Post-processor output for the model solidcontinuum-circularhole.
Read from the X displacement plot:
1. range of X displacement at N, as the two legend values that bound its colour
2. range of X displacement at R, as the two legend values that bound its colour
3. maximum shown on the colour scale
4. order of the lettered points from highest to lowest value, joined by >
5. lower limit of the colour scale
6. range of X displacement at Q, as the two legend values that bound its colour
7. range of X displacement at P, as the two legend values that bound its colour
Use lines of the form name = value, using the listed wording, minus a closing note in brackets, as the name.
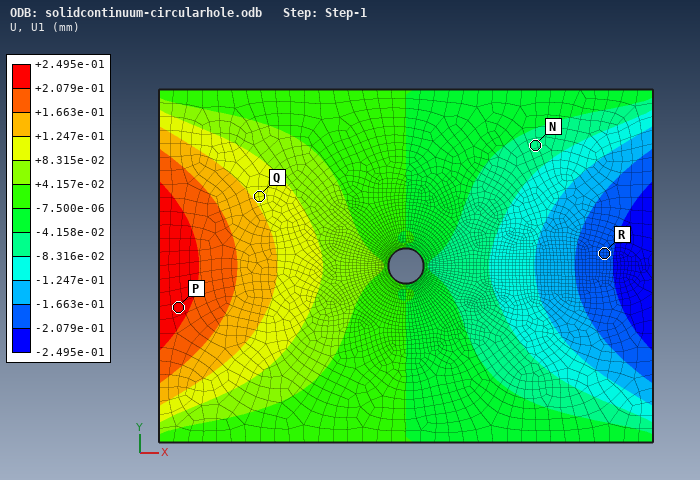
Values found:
range of X displacement at N, as the two legend values that bound its colour = -8.316e-02 to -4.158e-02 mm
range of X displacement at R, as the two legend values that bound its colour = -2.079e-01 to -1.663e-01 mm
maximum shown on the colour scale = +2.495e-01 mm
order of the lettered points from highest to lowest value, joined by > = P > Q > N > R
lower limit of the colour scale = -2.495e-01 mm
range of X displacement at Q, as the two legend values that bound its colour = +8.315e-02 to +1.247e-01 mm
range of X displacement at P, as the two legend values that bound its colour = +2.079e-01 to +2.495e-01 mm
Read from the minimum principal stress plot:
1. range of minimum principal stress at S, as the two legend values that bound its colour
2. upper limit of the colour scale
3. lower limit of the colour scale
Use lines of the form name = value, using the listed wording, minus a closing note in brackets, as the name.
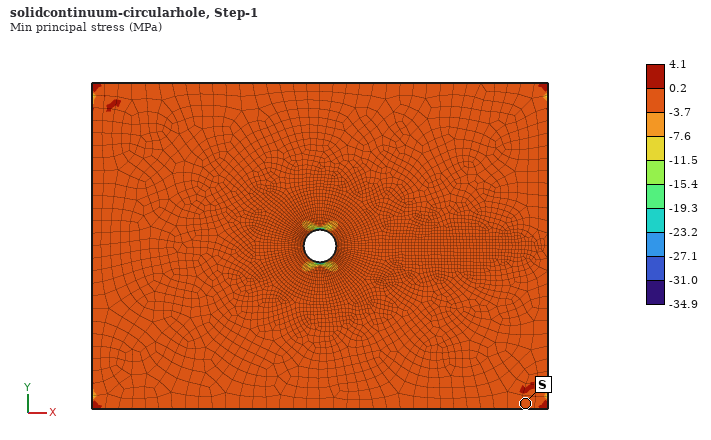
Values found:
range of minimum principal stress at S, as the two legend values that bound its colour = -3.7 to 0.2 MPa
upper limit of the colour scale = 4.1 MPa
lower limit of the colour scale = -34.9 MPa
